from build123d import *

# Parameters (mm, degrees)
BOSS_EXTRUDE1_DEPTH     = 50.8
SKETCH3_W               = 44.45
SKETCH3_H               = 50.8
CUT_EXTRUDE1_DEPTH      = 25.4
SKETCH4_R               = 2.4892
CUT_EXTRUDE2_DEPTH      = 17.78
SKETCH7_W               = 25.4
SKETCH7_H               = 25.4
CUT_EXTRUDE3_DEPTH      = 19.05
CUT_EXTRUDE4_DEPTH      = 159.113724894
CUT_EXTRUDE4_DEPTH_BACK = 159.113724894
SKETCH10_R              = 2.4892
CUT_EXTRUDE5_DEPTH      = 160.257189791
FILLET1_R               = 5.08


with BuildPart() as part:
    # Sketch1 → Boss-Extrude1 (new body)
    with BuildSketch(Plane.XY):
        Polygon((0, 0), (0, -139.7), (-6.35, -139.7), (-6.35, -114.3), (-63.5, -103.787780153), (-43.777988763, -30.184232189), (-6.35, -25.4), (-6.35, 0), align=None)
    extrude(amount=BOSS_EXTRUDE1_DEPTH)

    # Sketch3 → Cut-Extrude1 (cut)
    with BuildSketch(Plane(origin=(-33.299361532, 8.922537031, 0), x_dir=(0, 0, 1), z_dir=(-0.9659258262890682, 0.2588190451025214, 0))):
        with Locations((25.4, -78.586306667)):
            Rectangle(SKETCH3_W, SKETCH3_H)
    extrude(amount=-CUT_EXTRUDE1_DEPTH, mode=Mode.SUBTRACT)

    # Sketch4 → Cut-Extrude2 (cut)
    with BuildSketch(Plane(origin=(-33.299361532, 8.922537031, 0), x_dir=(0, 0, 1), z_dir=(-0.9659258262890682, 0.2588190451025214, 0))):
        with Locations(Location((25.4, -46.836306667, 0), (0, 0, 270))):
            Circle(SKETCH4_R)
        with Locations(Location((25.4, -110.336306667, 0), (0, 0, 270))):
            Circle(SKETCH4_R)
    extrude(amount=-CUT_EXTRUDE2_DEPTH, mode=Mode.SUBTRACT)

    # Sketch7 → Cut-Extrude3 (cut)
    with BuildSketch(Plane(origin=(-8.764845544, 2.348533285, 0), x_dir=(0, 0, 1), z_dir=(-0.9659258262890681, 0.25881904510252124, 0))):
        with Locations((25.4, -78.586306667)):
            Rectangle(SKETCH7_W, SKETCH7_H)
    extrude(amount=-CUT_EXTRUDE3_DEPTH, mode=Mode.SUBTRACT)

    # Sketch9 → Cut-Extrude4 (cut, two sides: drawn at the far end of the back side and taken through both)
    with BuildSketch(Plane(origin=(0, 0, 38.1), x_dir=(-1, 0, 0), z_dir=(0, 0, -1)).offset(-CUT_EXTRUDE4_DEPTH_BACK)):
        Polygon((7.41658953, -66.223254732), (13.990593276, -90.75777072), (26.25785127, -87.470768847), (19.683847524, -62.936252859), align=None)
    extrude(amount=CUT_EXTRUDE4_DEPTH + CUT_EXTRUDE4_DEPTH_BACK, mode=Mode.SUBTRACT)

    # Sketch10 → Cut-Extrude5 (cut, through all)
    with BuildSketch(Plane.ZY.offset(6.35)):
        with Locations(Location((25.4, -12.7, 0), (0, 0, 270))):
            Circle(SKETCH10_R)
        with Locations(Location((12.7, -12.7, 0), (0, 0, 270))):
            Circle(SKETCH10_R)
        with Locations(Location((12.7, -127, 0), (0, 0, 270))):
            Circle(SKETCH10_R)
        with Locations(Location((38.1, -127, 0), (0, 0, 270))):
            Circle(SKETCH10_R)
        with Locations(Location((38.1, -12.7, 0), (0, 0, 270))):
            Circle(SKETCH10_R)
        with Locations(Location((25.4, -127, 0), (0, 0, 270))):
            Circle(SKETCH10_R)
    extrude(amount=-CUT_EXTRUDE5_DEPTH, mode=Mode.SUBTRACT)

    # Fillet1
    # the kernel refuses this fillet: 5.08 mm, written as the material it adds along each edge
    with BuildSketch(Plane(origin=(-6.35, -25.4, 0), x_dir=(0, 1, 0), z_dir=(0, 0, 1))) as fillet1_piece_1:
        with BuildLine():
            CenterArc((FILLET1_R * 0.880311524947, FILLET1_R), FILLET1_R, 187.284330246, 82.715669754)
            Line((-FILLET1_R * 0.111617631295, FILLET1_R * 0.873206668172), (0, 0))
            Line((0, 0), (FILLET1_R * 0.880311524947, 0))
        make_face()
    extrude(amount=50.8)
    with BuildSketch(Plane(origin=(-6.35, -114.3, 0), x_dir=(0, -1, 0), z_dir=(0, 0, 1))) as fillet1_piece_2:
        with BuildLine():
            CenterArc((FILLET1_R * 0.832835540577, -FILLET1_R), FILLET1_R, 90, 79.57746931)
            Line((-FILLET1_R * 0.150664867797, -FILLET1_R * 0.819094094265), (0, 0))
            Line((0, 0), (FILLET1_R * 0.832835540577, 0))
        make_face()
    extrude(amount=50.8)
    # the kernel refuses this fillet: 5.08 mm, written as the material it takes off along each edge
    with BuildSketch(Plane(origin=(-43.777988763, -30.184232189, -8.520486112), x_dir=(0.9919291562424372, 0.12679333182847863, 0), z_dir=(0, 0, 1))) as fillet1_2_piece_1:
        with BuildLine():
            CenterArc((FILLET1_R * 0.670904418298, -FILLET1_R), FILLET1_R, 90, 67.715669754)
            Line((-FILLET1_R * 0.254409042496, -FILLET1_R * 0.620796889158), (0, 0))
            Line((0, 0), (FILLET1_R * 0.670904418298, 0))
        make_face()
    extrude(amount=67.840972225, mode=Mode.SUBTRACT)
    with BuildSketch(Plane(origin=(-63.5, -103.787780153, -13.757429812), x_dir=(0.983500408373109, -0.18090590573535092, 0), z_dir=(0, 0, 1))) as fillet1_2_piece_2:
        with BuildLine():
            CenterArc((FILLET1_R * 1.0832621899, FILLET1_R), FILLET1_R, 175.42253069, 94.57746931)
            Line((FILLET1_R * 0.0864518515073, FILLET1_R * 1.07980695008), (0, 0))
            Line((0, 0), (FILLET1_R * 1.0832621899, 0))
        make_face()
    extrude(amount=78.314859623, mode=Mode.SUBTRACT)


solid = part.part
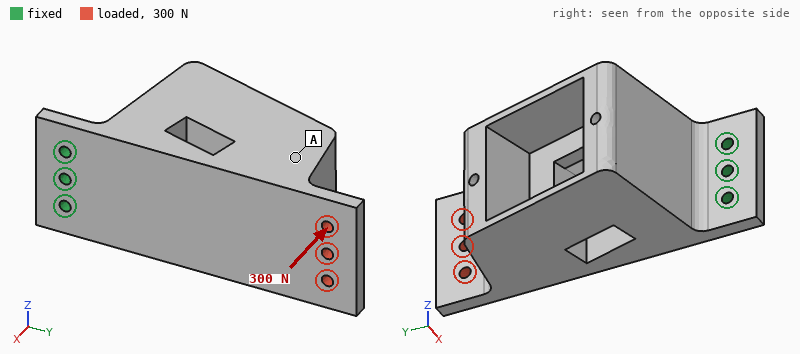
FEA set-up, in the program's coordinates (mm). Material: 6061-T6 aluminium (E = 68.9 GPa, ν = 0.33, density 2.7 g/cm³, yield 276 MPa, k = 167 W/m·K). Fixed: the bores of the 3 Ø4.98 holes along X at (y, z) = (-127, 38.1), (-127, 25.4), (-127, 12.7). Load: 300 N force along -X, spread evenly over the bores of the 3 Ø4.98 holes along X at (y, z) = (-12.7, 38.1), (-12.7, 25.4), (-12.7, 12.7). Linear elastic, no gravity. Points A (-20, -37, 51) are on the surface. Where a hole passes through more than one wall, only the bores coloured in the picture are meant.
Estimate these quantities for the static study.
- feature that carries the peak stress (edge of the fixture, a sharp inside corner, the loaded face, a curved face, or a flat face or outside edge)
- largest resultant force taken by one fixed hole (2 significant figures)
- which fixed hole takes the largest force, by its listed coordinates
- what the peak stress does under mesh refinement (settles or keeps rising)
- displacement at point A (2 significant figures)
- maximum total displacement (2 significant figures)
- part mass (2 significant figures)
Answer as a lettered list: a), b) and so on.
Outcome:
a) edge of the fixture
b) 250 N
c) (-127, 25.4)
d) keeps rising
e) 0.49 mm
f) 0.70 mm
g) 440 g
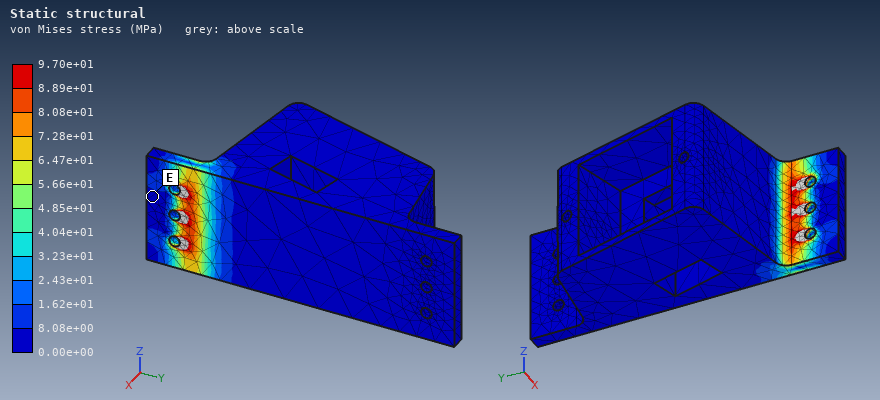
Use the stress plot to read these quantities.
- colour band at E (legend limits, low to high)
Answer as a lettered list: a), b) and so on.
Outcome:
a) 0.00e+00 to 8.08e+00 MPa
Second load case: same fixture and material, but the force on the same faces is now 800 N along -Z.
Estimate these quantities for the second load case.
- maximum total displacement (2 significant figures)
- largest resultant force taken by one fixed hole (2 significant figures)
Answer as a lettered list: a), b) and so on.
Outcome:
a) 0.10 mm
b) 3.2 kN
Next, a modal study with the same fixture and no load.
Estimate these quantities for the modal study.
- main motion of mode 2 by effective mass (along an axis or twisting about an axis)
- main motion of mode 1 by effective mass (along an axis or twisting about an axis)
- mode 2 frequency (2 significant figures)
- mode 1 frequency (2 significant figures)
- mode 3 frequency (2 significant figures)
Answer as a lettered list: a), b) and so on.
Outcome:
a) along Z
b) along X
c) 1300 Hz
d) 290 Hz
e) 1700 Hz
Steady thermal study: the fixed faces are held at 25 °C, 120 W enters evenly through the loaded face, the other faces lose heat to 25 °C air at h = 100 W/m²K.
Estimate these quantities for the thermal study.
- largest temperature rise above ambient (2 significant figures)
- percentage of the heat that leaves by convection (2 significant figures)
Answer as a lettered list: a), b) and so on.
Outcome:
a) 80 K
b) 71 %
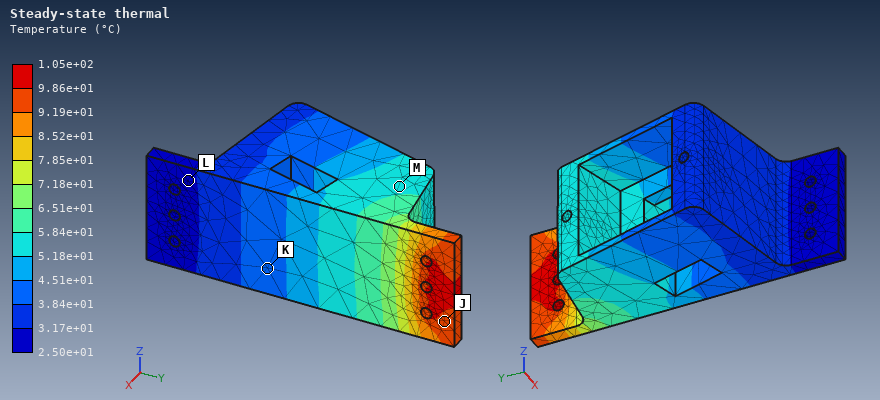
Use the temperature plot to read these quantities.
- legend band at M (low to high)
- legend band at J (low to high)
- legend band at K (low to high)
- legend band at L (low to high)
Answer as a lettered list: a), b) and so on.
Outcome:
a) 5.18e+01 to 5.84e+01 °C
b) 9.19e+01 to 9.86e+01 °C
c) 3.84e+01 to 4.51e+01 °C
d) 2.50e+01 to 3.17e+01 °C
